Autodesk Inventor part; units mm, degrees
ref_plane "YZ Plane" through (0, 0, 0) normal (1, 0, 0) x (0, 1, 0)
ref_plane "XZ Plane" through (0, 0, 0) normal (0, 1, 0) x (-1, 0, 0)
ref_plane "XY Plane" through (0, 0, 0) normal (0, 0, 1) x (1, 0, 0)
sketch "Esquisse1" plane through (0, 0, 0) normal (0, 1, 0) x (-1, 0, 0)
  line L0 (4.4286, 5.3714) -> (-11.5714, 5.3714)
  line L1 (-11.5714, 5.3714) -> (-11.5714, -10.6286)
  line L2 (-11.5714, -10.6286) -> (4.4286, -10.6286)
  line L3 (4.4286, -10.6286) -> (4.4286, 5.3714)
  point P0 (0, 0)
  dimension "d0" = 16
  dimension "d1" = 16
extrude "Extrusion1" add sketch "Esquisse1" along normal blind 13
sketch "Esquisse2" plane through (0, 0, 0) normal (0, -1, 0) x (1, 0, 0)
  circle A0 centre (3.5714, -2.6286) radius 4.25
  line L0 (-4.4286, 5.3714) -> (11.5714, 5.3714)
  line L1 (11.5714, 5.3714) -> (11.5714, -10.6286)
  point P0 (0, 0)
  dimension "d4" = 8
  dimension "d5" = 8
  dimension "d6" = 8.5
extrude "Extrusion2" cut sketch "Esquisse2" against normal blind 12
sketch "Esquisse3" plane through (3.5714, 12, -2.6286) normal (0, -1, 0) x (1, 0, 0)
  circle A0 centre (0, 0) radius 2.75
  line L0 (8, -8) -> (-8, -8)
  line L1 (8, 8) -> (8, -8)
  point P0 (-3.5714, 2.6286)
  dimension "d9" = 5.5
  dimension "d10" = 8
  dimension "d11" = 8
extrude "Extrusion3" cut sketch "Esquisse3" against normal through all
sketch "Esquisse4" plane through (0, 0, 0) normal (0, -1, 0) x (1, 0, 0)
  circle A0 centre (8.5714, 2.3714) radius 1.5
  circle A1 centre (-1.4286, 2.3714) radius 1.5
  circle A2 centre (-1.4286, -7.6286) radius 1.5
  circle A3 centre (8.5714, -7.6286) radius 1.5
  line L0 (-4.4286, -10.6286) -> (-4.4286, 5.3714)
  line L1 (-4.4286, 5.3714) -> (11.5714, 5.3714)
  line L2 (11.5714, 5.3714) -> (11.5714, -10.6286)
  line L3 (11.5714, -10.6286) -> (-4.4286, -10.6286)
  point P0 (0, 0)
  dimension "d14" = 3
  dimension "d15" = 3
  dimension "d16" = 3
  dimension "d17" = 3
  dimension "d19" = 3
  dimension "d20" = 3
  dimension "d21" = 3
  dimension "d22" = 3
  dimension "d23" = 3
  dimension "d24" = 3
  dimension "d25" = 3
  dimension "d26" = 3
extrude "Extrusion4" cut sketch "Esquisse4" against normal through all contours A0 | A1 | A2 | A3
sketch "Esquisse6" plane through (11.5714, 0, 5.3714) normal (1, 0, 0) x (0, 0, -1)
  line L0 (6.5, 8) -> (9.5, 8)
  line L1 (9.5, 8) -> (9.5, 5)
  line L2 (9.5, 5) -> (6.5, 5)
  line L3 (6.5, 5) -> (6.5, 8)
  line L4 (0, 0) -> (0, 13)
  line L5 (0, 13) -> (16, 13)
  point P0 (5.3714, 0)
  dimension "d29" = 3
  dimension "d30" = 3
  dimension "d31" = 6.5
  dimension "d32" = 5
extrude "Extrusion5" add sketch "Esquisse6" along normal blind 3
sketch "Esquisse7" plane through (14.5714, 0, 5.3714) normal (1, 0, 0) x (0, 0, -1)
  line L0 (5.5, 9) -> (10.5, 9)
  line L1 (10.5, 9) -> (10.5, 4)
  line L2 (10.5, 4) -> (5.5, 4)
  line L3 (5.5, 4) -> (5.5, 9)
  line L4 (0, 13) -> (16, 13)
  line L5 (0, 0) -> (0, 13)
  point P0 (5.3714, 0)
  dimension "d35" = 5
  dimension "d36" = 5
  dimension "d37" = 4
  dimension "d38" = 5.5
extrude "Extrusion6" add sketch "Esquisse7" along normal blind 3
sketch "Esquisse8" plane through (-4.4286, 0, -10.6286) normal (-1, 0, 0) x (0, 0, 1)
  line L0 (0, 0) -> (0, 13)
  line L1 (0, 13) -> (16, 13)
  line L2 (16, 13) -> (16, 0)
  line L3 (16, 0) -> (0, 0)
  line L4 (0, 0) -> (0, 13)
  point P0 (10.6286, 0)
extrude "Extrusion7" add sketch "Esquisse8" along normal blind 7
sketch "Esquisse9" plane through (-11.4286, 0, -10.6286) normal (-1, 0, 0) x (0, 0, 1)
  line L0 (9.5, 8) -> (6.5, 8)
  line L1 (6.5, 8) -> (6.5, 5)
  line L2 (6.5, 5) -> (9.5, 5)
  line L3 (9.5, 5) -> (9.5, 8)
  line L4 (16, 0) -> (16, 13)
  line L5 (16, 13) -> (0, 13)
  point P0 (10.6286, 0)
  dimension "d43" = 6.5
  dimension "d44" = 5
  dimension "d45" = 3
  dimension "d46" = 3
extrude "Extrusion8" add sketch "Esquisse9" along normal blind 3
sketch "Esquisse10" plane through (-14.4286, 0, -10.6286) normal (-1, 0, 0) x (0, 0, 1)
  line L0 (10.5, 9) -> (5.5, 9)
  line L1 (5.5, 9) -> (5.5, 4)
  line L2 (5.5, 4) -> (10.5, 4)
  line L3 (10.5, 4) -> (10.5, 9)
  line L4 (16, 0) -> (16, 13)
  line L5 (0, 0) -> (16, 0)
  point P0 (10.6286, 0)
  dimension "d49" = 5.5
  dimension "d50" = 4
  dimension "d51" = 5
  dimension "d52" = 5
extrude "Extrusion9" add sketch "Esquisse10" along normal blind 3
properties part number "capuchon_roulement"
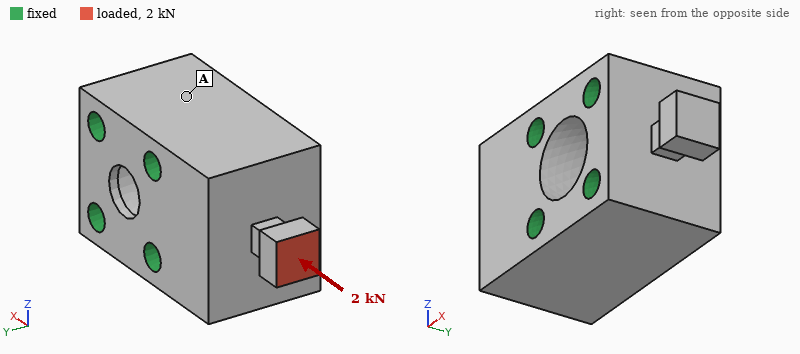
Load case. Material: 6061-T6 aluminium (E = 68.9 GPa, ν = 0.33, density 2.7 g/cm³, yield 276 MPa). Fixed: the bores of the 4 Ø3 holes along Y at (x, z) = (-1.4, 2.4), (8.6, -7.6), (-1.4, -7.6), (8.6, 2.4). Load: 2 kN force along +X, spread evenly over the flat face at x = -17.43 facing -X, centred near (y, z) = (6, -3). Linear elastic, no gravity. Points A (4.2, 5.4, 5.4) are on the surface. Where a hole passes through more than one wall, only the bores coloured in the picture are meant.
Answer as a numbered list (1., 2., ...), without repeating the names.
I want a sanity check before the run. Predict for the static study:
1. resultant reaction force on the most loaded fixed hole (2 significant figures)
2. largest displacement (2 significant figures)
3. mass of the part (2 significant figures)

1. 1.1 kN
2. 22 µm
3. 11 g
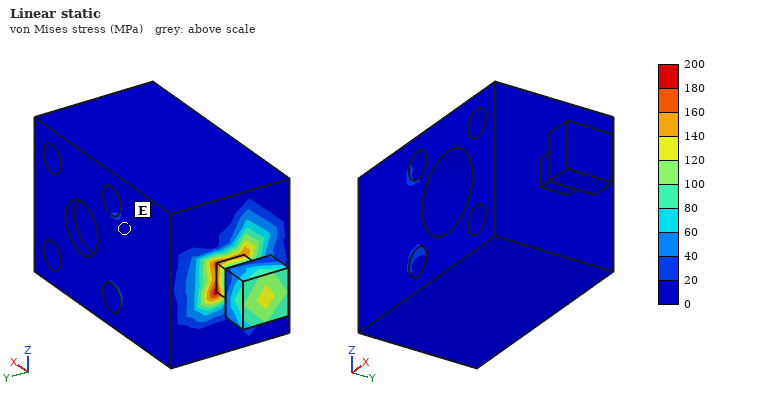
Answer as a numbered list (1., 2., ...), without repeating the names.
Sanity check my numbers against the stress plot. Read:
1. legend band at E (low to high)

1. 0 to 20 MPa
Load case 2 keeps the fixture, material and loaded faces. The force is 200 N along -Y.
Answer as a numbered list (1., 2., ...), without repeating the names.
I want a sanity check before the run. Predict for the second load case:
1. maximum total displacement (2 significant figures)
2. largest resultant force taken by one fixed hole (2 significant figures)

1. 49 µm
2. 100 N
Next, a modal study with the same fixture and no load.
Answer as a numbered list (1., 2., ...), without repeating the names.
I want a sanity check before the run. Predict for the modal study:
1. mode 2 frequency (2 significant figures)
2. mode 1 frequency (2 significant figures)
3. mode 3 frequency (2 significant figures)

1. 30 kHz
2. 29 kHz
3. 30 kHz
